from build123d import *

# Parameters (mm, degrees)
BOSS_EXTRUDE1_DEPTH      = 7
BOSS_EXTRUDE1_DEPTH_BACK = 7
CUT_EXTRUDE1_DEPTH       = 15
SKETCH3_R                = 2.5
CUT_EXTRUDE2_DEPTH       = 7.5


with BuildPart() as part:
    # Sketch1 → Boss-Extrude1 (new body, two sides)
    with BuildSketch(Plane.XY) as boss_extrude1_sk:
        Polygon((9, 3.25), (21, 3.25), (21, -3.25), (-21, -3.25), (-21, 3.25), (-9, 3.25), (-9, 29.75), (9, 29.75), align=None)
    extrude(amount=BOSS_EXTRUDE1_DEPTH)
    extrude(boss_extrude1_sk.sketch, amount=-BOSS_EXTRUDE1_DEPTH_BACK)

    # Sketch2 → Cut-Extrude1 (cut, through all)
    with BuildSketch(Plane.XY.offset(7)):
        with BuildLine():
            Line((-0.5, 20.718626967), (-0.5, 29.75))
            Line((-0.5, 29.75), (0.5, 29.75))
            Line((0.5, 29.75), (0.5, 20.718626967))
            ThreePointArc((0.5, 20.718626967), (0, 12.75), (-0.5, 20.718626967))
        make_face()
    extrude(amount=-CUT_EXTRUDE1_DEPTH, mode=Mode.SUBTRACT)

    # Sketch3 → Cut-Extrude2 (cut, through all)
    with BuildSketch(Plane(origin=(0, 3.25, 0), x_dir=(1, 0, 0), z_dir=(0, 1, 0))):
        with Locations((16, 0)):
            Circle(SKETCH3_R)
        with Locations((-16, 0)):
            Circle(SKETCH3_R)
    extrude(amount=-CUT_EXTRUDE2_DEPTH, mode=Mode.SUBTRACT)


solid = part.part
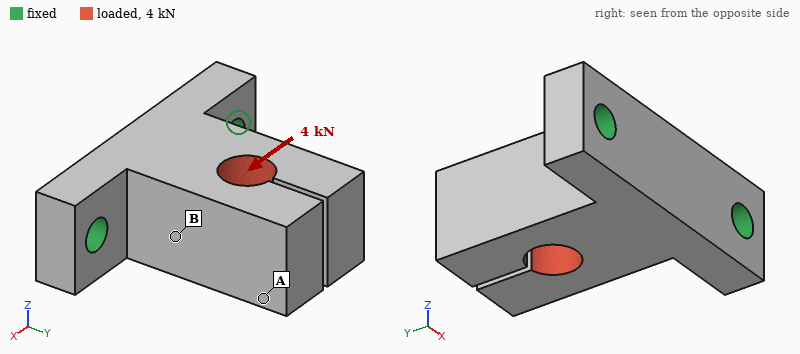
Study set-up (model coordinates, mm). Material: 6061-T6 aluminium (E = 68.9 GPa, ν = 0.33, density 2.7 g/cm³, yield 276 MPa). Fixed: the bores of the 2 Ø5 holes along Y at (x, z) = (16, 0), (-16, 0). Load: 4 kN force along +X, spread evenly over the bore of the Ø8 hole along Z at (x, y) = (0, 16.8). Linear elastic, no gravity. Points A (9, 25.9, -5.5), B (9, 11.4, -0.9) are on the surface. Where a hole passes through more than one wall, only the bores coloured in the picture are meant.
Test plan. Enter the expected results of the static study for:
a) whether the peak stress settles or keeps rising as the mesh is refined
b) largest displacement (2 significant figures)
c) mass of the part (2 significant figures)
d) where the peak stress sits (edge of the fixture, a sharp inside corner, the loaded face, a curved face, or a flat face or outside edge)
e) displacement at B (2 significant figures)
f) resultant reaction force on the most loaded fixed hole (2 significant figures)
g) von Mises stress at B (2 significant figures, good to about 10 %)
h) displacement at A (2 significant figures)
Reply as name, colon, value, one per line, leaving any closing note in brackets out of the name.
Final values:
whether the peak stress settles or keeps rising as the mesh is refined: keeps rising
largest displacement: 0.11 mm
mass of the part: 25 g
where the peak stress sits: edge of the fixture
displacement at B: 0.035 mm
resultant reaction force on the most loaded fixed hole: 3.4 kN
von Mises stress at B: 61 MPa
displacement at A: 0.096 mm
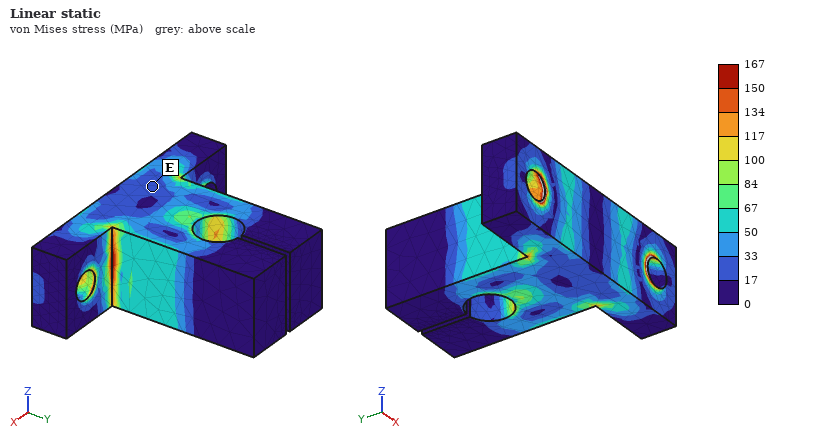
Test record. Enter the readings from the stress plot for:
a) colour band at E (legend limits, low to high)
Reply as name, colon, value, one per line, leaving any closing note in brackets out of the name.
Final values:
colour band at E: 17 to 33 MPa
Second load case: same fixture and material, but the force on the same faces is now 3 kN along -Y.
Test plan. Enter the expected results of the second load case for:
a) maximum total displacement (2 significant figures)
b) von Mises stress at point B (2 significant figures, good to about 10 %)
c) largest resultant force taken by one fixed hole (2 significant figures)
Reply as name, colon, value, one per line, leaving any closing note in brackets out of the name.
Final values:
maximum total displacement: 40 µm
von Mises stress at point B: 12 MPa
largest resultant force taken by one fixed hole: 1.6 kN
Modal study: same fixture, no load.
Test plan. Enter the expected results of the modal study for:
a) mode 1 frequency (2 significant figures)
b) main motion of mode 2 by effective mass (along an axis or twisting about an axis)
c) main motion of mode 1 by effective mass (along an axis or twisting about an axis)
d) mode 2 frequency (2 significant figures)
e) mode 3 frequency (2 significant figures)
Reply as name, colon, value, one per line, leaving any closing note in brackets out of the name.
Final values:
mode 1 frequency: 5100 Hz
main motion of mode 2 by effective mass: along X
main motion of mode 1 by effective mass: along Z
mode 2 frequency: 7800 Hz
mode 3 frequency: 9300 Hz
